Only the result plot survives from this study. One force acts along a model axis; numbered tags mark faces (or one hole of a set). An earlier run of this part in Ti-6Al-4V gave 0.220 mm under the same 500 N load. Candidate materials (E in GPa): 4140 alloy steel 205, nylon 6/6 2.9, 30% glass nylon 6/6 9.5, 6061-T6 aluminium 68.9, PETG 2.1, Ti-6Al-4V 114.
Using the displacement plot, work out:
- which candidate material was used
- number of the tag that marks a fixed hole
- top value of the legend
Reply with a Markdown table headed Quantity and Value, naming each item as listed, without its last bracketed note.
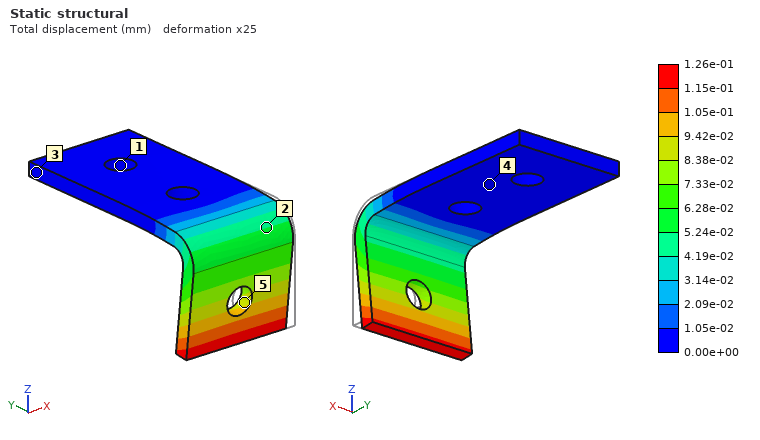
| Quantity | Value |
|---|---|
| which candidate material was used | 4140 alloy steel |
| number of the tag that marks a fixed hole | 1 |
| top value of the legend | 1.26e-01 mm |
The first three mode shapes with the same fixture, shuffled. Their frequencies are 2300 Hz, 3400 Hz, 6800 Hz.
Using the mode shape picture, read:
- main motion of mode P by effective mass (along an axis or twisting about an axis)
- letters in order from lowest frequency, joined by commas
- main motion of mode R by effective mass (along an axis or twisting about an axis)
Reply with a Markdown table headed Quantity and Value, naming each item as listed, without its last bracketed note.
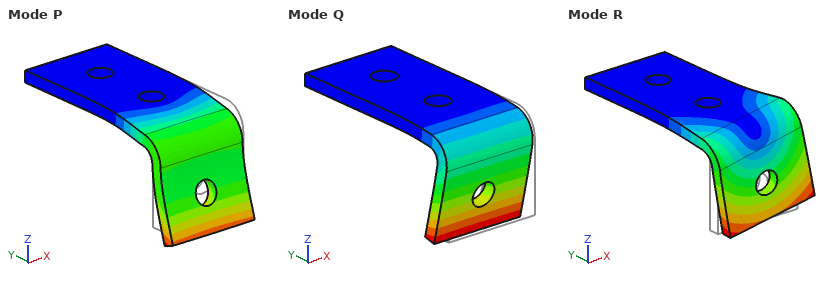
| Quantity | Value |
|---|---|
| main motion of mode P by effective mass | along Z |
| letters in order from lowest frequency, joined by commas | Q, R, P |
| main motion of mode R by effective mass | along X |
